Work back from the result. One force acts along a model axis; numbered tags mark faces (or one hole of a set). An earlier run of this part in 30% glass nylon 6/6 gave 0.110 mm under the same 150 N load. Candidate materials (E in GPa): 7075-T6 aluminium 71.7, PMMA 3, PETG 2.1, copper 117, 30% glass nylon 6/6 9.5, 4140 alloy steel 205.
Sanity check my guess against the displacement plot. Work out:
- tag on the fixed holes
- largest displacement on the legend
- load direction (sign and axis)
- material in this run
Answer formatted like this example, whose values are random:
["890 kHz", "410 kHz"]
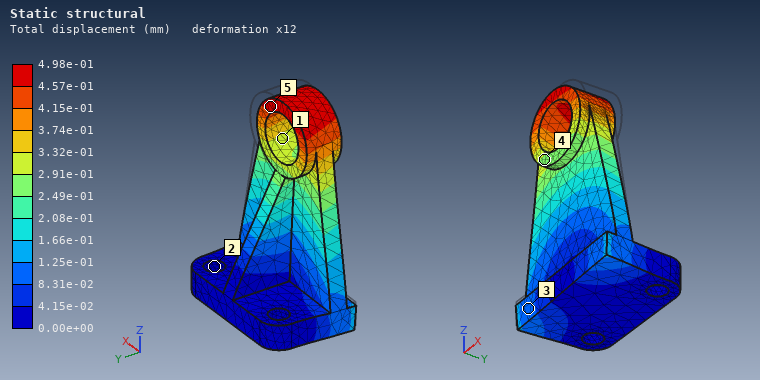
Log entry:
["2", "4.98e-01 mm", "-X", "PETG"]
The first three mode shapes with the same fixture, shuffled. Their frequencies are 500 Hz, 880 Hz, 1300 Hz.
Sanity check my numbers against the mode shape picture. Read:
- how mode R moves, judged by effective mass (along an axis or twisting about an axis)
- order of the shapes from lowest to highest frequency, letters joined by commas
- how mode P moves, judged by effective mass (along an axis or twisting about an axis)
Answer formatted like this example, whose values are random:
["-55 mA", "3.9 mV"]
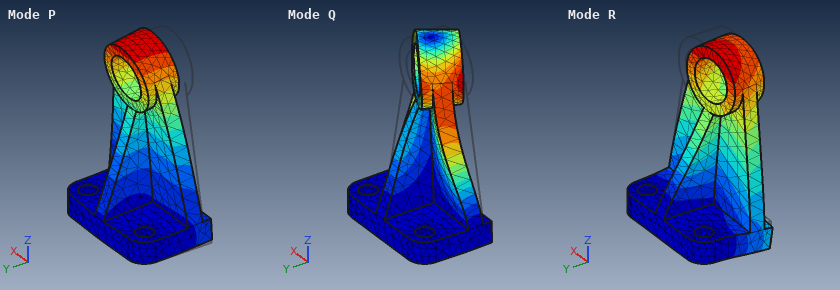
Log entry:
["along X", "P, R, Q", "along Y"]
